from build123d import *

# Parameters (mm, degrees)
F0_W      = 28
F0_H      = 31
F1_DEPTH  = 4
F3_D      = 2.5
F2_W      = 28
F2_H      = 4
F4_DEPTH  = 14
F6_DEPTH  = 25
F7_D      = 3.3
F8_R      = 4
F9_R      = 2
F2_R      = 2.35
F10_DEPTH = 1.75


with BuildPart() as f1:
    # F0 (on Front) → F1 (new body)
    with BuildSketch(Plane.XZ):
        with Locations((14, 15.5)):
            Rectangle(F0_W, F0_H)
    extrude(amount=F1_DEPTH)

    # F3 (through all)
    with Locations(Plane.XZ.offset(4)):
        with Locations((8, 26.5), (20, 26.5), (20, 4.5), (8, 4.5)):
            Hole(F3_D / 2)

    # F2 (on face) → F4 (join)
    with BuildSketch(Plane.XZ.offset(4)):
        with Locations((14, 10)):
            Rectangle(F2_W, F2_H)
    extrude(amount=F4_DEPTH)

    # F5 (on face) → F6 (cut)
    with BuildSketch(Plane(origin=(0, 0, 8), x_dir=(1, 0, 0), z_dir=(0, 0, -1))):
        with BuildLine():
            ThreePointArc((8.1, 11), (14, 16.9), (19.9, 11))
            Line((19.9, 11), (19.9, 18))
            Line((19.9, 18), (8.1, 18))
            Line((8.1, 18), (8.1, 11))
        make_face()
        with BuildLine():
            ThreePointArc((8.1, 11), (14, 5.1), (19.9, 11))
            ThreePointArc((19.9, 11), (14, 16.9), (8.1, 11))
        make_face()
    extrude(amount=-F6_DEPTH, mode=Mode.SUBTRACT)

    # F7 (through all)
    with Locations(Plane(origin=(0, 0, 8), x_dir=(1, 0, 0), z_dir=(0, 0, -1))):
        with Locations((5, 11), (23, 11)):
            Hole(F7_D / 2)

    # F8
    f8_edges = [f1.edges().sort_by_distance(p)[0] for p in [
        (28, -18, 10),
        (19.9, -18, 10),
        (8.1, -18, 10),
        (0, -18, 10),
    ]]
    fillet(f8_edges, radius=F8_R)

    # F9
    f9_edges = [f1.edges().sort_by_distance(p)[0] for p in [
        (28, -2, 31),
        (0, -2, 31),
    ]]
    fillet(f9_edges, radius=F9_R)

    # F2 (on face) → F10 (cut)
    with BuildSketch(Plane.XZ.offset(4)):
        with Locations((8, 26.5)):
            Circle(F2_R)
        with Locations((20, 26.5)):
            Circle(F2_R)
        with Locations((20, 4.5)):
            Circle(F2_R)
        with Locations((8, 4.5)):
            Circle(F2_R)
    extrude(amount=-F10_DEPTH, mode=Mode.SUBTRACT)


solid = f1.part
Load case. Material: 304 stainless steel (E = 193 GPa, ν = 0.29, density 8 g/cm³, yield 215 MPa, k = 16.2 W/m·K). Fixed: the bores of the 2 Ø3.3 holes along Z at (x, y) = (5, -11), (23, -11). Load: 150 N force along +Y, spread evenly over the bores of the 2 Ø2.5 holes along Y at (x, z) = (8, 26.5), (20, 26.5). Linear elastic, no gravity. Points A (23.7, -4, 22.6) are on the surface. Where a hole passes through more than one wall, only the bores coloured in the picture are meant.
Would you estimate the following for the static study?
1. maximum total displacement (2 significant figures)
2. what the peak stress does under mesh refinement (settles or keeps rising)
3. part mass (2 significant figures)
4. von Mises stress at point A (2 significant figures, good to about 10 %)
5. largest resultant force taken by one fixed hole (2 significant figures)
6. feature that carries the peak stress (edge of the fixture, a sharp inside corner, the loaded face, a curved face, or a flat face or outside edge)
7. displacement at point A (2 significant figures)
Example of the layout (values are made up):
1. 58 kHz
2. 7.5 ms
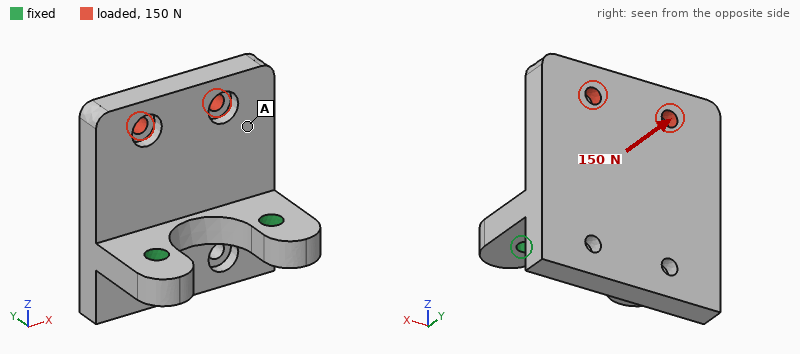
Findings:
1. 31 µm
2. keeps rising
3. 34 g
4. 9.0 MPa
5. 83 N
6. edge of the fixture
7. 16 µm
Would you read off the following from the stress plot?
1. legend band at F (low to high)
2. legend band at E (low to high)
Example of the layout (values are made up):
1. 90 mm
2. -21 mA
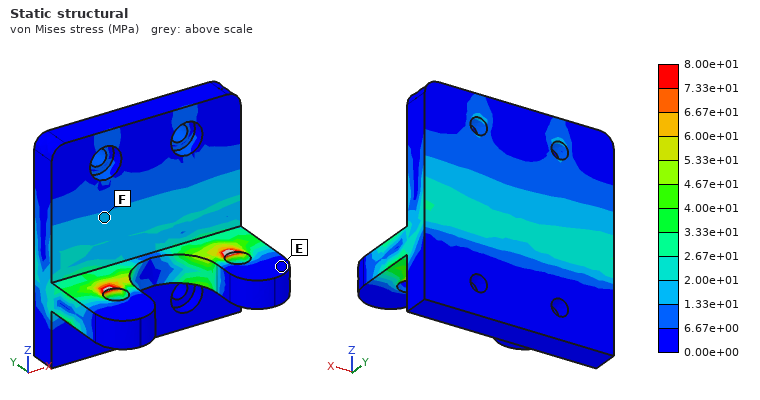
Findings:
1. 1.33e+01 to 2.00e+01 MPa
2. 0.00e+00 to 6.67e+00 MPa
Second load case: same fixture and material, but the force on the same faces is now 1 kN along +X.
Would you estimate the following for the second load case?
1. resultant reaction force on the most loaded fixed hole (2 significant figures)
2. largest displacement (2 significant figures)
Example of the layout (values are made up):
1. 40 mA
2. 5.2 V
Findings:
1. 980 N
2. 26 µm
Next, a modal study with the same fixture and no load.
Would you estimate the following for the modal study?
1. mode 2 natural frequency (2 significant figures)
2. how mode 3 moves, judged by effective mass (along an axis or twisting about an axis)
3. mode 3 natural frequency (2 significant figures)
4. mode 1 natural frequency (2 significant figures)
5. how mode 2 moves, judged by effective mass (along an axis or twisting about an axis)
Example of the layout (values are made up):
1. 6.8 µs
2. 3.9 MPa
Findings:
1. 9100 Hz
2. along Z
3. 13 kHz
4. 3900 Hz
5. along X
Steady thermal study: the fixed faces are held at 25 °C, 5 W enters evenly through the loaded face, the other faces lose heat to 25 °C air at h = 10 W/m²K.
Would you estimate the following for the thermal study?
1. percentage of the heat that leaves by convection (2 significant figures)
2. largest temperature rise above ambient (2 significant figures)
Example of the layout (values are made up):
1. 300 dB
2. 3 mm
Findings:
1. 19 %
2. 77 K
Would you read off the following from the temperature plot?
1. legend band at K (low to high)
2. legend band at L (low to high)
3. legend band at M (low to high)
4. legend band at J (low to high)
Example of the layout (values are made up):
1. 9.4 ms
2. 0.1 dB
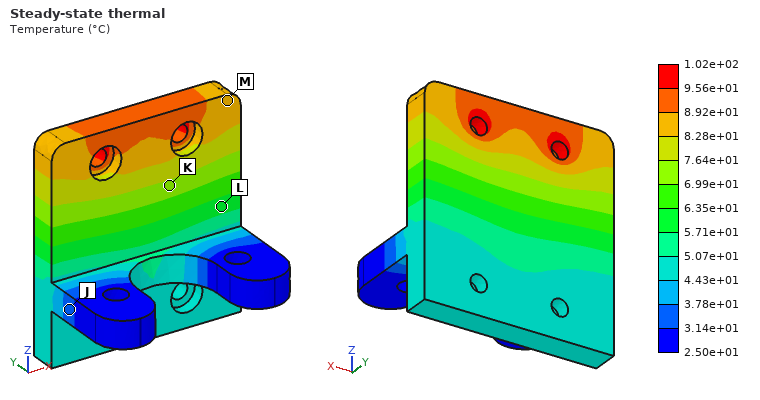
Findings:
1. 6.99e+01 to 7.64e+01 °C
2. 5.71e+01 to 6.35e+01 °C
3. 8.28e+01 to 8.92e+01 °C
4. 3.14e+01 to 3.78e+01 °C
